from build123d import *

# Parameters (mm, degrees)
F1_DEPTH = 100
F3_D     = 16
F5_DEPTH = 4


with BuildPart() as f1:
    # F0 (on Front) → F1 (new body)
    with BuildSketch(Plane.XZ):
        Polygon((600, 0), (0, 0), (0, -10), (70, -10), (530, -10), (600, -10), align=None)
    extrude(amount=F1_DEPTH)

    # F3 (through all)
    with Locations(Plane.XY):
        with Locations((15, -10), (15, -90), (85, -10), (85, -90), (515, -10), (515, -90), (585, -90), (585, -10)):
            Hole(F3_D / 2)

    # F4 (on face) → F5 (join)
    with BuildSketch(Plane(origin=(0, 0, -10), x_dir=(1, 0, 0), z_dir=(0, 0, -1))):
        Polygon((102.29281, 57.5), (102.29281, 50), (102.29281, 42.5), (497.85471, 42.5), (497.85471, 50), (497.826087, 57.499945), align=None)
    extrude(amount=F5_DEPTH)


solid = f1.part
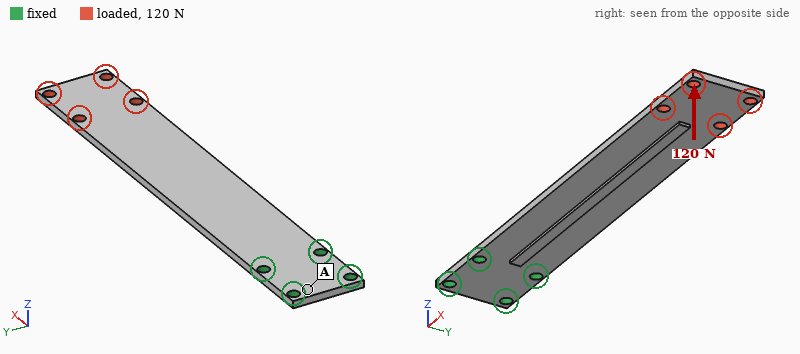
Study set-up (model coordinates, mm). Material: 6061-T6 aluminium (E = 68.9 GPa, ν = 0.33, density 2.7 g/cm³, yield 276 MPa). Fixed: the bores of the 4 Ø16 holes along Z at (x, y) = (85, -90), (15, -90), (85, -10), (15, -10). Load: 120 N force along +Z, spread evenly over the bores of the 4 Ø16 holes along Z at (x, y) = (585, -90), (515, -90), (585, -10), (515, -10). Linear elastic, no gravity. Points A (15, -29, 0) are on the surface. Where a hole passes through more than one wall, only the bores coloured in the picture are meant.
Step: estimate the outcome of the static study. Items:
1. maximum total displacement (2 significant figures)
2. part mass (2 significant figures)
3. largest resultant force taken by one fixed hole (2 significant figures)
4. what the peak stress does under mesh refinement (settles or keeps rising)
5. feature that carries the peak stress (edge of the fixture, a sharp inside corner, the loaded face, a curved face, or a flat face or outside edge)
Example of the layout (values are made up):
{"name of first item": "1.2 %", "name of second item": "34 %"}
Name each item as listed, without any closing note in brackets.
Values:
{"maximum total displacement": "6.3 mm", "part mass": "1.6 kg", "largest resultant force taken by one fixed hole": "170 N", "what the peak stress does under mesh refinement": "keeps rising", "feature that carries the peak stress": "edge of the fixture"}
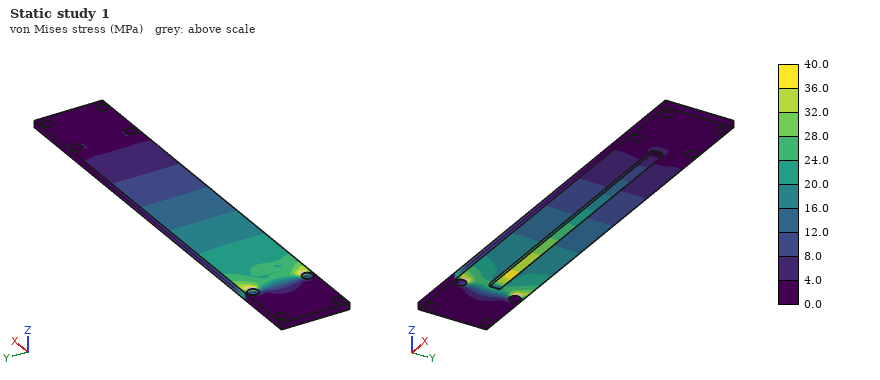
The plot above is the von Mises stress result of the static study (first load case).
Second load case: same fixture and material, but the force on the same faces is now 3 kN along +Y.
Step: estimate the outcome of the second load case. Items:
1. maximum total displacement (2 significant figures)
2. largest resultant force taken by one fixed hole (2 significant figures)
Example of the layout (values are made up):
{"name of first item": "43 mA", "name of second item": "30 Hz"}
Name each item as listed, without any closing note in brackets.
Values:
{"maximum total displacement": "2.1 mm", "largest resultant force taken by one fixed hole": "17 kN"}
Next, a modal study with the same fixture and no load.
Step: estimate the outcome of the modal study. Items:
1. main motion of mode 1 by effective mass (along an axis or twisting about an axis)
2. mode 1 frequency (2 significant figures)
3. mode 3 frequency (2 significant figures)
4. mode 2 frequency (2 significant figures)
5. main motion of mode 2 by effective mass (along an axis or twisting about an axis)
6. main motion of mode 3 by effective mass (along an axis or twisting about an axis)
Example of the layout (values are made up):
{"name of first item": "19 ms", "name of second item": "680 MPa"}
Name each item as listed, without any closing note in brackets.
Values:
{"main motion of mode 1 by effective mass": "along Z", "mode 1 frequency": "35 Hz", "mode 3 frequency": "310 Hz", "mode 2 frequency": "220 Hz", "main motion of mode 2 by effective mass": "along Z", "main motion of mode 3 by effective mass": "along Y"}
